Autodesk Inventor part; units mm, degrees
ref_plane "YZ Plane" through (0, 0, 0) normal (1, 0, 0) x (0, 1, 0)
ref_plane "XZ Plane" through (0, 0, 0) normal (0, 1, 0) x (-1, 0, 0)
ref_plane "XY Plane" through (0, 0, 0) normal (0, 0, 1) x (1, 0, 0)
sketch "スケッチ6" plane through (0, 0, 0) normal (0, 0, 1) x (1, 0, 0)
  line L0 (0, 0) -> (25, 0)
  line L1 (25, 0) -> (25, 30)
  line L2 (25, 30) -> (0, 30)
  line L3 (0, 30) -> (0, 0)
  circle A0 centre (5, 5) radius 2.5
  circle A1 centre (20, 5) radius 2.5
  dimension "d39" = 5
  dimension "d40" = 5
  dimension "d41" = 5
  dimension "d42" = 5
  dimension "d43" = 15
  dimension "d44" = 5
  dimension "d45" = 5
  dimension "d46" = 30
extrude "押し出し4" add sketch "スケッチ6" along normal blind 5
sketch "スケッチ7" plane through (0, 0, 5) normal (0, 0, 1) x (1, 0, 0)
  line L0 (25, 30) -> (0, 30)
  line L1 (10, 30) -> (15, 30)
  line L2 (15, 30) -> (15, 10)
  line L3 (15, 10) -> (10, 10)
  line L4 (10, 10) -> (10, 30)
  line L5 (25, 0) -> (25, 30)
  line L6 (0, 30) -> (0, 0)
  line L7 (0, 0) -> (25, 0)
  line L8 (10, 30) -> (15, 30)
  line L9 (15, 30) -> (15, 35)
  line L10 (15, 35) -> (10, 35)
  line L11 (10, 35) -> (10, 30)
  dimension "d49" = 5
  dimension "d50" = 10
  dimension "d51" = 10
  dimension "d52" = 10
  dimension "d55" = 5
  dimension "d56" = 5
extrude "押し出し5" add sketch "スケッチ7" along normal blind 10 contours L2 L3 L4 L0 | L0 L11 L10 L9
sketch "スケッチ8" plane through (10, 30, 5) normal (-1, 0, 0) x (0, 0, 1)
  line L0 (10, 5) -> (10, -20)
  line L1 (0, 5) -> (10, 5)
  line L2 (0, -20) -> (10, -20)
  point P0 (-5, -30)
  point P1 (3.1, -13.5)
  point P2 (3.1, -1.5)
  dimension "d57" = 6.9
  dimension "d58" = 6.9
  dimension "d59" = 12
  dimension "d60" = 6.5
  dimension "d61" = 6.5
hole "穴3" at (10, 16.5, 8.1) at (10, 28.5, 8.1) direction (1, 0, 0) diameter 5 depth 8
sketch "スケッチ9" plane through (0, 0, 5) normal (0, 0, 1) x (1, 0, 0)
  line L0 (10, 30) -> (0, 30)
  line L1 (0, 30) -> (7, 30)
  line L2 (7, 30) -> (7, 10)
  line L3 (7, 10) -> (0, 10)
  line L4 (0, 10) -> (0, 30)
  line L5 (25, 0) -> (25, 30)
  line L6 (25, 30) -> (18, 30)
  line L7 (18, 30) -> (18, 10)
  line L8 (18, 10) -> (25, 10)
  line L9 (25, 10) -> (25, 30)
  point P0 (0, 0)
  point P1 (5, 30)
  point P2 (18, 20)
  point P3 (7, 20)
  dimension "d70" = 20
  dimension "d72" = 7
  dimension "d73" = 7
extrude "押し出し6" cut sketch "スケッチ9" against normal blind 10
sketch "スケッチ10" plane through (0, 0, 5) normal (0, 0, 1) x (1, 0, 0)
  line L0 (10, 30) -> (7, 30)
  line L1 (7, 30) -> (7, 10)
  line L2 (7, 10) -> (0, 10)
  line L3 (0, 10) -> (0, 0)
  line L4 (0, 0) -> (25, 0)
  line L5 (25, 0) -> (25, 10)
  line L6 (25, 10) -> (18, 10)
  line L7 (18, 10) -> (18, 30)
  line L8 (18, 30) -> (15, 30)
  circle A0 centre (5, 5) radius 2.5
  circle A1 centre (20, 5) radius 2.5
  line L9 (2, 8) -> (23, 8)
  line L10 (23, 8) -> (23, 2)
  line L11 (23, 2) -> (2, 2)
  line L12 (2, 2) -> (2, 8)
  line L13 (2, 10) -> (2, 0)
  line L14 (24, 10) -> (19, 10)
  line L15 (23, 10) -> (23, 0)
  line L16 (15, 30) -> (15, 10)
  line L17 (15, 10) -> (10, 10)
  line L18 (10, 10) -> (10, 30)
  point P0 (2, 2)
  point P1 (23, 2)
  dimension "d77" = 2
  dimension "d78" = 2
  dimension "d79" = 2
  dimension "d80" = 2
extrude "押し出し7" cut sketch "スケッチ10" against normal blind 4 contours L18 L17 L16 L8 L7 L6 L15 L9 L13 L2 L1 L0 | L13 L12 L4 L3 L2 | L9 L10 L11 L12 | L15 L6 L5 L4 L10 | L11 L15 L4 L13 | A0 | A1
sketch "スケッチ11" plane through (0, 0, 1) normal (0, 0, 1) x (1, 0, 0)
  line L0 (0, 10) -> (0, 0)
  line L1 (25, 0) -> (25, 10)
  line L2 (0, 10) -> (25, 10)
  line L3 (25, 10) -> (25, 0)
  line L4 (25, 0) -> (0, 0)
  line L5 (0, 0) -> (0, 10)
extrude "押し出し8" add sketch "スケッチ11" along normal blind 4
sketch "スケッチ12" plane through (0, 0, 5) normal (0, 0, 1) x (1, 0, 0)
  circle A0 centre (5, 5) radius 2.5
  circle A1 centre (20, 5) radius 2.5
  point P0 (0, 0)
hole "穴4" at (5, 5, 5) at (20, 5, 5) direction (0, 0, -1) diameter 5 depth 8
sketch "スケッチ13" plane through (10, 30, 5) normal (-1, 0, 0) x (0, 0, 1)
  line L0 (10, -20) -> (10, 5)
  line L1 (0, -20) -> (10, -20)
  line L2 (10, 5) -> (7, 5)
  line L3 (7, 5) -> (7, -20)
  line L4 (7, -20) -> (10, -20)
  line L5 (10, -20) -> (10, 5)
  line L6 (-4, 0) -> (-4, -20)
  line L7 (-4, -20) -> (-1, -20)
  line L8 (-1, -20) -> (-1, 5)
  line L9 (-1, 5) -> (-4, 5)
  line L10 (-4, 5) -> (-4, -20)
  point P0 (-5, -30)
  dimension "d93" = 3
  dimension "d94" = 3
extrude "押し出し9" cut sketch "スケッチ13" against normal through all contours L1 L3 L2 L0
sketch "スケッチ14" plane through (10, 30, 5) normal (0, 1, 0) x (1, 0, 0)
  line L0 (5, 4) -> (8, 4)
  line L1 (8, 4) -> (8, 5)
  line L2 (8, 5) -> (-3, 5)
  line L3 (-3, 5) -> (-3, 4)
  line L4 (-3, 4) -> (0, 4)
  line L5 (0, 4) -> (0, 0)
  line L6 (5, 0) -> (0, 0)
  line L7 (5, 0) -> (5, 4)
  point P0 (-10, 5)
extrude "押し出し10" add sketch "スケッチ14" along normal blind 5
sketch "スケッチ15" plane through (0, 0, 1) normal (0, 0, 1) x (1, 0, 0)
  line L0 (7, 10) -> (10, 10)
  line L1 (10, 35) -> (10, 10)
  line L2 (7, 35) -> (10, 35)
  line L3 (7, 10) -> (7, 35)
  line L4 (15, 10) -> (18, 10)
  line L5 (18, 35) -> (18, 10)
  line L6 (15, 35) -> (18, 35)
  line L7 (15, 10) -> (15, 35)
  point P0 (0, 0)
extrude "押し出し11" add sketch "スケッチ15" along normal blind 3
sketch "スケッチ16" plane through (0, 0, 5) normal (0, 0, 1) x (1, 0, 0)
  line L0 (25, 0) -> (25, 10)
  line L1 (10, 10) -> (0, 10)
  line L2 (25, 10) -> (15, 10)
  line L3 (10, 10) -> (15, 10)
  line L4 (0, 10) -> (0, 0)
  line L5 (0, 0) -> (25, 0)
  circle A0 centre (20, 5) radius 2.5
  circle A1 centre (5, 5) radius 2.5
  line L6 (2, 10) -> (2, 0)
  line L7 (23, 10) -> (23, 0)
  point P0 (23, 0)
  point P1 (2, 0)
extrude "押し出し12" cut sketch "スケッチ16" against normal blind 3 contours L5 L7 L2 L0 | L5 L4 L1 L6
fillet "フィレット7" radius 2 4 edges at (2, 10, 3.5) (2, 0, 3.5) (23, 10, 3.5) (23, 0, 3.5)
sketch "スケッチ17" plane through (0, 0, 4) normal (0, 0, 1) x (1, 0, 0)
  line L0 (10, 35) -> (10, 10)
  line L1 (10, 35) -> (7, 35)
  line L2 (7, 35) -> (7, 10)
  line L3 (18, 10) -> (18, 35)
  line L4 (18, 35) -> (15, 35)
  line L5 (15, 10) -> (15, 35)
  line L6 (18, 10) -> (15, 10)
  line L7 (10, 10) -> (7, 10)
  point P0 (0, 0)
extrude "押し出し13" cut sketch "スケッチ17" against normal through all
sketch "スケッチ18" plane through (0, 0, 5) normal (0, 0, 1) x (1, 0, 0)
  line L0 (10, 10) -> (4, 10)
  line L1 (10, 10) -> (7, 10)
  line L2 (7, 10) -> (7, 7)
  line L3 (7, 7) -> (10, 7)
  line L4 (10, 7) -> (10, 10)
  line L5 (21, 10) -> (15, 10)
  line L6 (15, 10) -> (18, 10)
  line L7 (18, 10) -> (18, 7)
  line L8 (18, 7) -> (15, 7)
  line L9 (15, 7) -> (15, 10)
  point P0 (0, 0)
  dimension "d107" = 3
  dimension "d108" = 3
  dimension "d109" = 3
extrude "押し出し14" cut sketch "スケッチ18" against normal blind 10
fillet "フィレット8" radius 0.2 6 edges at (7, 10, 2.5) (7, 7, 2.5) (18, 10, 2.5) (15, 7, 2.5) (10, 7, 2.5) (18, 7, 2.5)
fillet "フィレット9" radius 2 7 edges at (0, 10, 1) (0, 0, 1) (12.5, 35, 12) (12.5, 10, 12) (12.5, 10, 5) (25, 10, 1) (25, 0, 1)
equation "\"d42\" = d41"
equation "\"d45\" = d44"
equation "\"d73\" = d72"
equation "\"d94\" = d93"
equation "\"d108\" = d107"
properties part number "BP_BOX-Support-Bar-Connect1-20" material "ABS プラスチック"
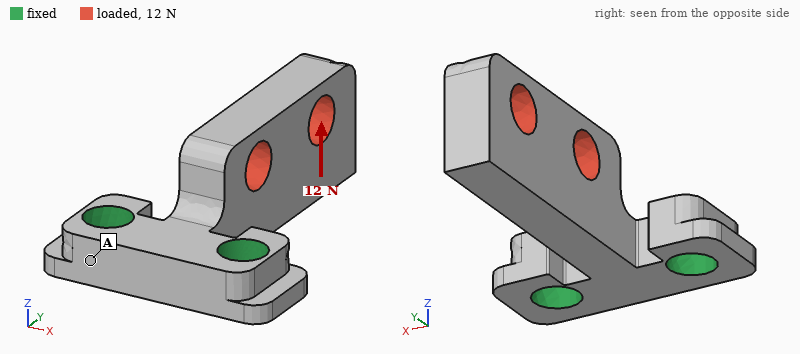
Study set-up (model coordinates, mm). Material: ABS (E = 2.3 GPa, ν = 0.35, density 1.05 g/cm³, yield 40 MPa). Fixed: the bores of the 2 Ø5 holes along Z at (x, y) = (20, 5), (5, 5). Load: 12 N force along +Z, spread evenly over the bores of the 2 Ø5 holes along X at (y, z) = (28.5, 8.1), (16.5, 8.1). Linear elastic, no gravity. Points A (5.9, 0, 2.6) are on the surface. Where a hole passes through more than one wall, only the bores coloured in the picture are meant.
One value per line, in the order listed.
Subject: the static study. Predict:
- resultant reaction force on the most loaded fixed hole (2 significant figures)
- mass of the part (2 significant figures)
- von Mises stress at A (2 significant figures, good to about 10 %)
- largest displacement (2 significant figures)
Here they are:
6.0 N
2.2 g
1.4 MPa
0.38 mm
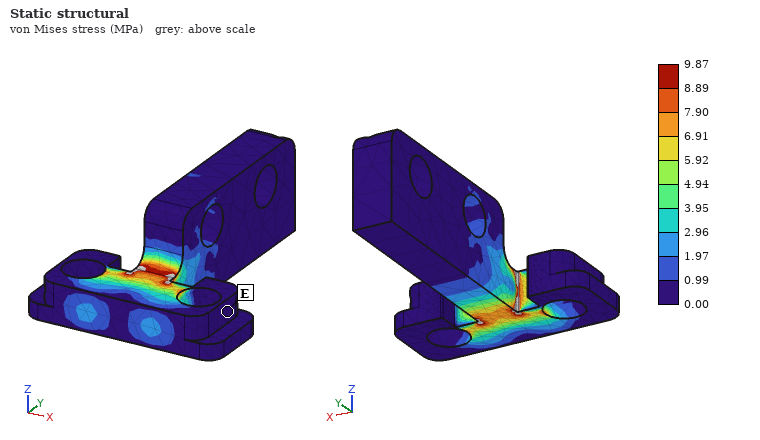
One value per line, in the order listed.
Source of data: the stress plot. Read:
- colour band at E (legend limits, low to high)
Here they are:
0.00 to 0.99 MPa
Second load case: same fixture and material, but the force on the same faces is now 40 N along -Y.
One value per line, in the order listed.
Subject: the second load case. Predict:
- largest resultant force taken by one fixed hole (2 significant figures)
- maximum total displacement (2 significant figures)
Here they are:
20 N
0.45 mm
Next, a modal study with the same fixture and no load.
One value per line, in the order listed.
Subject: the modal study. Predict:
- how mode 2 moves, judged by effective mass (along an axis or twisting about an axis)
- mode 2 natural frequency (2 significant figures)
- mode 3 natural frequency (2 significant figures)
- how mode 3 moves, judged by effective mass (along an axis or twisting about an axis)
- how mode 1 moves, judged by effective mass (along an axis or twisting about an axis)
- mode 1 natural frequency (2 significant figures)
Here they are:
along X
990 Hz
3300 Hz
twisting about Y
along Z
920 Hz
